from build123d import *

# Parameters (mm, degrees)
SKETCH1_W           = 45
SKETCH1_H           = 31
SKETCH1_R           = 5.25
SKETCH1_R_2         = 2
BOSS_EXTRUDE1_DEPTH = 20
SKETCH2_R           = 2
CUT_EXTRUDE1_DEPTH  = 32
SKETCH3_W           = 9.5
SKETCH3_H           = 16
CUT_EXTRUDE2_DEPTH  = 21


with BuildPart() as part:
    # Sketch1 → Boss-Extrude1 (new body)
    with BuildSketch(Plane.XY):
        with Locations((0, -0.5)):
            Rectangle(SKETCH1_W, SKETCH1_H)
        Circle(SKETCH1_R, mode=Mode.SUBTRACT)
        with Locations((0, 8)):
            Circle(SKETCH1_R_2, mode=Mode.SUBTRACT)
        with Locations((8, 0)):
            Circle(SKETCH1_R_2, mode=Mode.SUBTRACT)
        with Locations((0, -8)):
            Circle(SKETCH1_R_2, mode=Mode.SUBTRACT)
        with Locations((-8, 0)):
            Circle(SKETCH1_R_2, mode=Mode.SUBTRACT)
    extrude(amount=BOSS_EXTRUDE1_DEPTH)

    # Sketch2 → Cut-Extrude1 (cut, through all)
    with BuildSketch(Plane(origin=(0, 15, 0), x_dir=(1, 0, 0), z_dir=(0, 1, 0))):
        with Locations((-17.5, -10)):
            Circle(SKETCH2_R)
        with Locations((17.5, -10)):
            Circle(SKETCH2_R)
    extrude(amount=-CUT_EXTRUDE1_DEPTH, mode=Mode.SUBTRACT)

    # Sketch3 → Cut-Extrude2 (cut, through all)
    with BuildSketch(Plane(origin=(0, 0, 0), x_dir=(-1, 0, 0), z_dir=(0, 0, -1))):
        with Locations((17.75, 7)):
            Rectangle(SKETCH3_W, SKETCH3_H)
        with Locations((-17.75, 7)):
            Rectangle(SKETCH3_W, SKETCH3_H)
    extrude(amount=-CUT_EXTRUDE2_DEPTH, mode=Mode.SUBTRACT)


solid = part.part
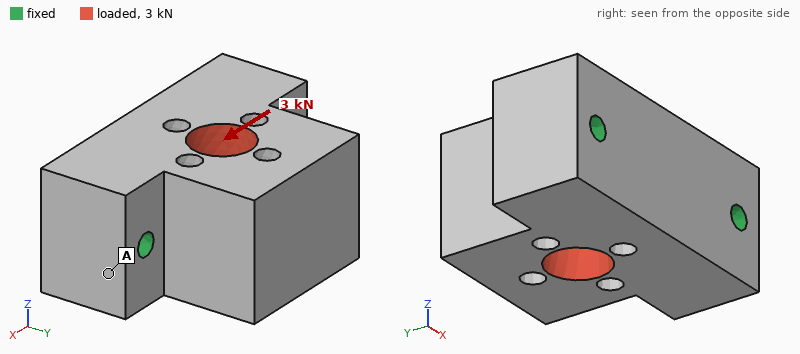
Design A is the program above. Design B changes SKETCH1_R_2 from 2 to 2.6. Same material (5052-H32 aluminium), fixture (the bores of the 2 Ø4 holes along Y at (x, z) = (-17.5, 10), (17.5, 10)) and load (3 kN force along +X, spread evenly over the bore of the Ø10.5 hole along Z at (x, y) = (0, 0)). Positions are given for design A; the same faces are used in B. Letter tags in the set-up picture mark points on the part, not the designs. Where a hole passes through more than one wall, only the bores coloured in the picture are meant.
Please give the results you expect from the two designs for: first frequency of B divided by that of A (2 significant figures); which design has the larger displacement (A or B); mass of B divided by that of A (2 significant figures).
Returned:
0.96
B
0.96
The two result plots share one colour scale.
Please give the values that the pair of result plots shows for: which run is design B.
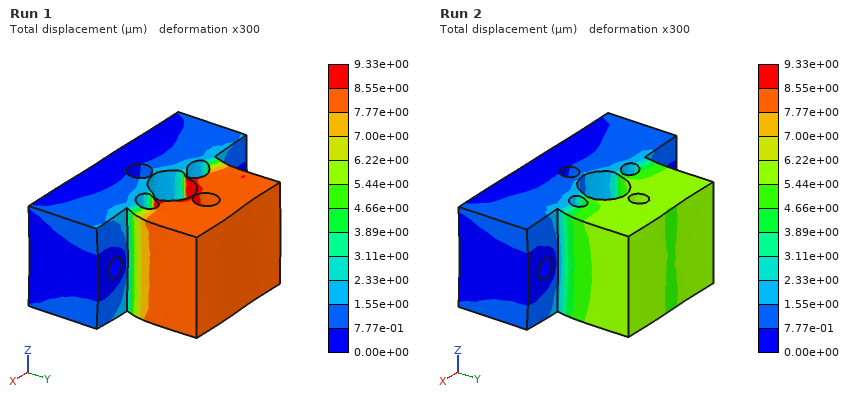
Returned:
Run 1
